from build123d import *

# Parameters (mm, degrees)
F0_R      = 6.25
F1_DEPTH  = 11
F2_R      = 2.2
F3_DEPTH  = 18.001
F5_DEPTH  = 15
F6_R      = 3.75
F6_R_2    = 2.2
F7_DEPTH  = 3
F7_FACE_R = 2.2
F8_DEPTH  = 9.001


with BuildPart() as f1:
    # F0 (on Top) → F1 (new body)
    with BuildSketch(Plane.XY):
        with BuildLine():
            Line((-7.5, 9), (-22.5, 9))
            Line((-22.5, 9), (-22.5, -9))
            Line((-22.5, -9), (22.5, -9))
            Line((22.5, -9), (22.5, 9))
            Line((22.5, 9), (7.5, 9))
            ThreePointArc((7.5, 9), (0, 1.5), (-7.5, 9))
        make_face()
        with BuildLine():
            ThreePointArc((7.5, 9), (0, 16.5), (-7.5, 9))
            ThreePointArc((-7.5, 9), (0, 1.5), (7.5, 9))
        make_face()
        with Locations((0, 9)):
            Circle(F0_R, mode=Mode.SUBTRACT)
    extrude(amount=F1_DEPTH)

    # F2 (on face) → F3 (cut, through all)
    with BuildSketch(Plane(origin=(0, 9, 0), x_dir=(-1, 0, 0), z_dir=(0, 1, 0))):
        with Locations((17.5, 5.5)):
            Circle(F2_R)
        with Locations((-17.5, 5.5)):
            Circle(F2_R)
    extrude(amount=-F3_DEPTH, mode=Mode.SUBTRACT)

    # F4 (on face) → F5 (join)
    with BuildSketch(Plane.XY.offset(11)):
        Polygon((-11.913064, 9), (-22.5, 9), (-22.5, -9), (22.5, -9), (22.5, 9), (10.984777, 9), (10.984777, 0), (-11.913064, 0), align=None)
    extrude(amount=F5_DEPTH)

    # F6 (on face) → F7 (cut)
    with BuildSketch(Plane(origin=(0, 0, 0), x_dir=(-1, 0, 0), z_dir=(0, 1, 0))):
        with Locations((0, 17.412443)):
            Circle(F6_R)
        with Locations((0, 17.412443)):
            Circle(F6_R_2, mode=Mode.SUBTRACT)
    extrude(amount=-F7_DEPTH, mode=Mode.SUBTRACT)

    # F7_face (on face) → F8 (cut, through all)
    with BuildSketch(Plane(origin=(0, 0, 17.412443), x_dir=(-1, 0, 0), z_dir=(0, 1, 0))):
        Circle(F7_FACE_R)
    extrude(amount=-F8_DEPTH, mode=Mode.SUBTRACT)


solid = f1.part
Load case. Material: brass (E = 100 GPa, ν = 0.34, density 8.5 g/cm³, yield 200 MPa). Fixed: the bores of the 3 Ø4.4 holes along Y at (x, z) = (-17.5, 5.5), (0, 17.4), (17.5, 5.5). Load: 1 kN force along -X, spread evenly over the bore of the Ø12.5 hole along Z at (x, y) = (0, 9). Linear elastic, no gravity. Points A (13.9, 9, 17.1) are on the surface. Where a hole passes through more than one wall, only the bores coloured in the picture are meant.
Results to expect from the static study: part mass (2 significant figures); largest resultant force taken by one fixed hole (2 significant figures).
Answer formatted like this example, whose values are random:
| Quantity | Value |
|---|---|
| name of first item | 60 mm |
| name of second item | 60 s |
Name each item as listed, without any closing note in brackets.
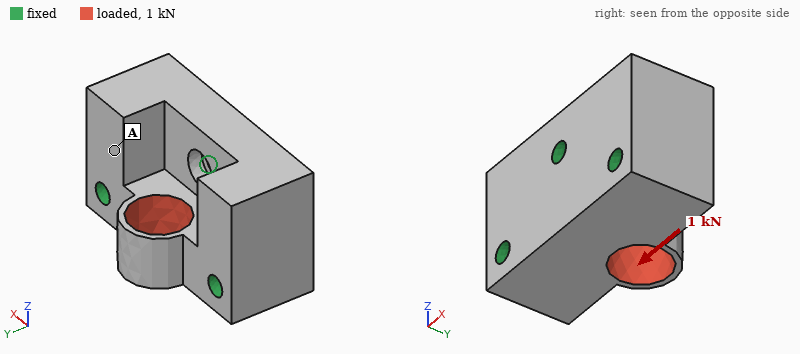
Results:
| Quantity | Value |
|---|---|
| part mass | 140 g |
| largest resultant force taken by one fixed hole | 510 N |
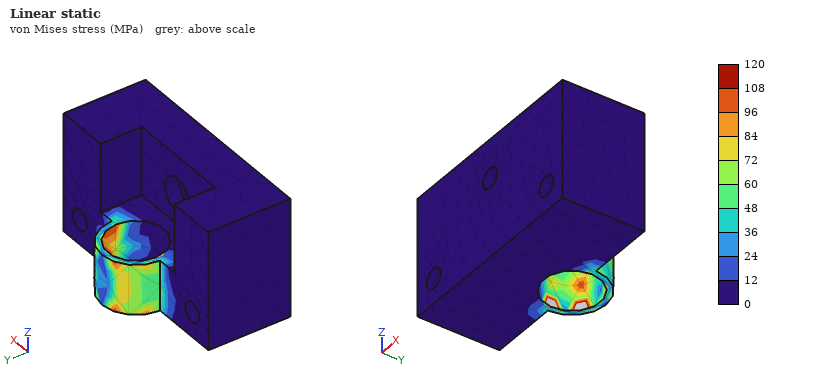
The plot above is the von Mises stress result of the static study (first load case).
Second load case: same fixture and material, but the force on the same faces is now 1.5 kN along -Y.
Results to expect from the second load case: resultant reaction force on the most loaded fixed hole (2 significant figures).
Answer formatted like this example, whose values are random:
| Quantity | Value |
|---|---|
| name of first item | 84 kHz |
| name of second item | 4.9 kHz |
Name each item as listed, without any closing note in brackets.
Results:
| Quantity | Value |
|---|---|
| resultant reaction force on the most loaded fixed hole | 620 N |
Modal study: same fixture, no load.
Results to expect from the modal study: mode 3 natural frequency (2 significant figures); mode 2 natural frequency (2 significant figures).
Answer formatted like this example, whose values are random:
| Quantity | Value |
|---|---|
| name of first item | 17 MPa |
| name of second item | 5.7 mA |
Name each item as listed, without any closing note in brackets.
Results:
| Quantity | Value |
|---|---|
| mode 3 natural frequency | 18 kHz |
| mode 2 natural frequency | 18 kHz |
